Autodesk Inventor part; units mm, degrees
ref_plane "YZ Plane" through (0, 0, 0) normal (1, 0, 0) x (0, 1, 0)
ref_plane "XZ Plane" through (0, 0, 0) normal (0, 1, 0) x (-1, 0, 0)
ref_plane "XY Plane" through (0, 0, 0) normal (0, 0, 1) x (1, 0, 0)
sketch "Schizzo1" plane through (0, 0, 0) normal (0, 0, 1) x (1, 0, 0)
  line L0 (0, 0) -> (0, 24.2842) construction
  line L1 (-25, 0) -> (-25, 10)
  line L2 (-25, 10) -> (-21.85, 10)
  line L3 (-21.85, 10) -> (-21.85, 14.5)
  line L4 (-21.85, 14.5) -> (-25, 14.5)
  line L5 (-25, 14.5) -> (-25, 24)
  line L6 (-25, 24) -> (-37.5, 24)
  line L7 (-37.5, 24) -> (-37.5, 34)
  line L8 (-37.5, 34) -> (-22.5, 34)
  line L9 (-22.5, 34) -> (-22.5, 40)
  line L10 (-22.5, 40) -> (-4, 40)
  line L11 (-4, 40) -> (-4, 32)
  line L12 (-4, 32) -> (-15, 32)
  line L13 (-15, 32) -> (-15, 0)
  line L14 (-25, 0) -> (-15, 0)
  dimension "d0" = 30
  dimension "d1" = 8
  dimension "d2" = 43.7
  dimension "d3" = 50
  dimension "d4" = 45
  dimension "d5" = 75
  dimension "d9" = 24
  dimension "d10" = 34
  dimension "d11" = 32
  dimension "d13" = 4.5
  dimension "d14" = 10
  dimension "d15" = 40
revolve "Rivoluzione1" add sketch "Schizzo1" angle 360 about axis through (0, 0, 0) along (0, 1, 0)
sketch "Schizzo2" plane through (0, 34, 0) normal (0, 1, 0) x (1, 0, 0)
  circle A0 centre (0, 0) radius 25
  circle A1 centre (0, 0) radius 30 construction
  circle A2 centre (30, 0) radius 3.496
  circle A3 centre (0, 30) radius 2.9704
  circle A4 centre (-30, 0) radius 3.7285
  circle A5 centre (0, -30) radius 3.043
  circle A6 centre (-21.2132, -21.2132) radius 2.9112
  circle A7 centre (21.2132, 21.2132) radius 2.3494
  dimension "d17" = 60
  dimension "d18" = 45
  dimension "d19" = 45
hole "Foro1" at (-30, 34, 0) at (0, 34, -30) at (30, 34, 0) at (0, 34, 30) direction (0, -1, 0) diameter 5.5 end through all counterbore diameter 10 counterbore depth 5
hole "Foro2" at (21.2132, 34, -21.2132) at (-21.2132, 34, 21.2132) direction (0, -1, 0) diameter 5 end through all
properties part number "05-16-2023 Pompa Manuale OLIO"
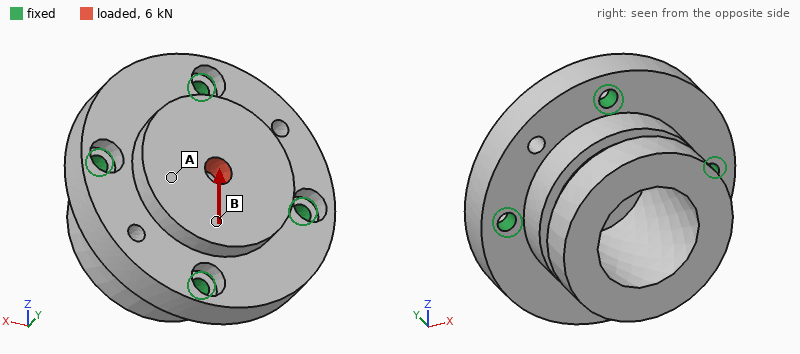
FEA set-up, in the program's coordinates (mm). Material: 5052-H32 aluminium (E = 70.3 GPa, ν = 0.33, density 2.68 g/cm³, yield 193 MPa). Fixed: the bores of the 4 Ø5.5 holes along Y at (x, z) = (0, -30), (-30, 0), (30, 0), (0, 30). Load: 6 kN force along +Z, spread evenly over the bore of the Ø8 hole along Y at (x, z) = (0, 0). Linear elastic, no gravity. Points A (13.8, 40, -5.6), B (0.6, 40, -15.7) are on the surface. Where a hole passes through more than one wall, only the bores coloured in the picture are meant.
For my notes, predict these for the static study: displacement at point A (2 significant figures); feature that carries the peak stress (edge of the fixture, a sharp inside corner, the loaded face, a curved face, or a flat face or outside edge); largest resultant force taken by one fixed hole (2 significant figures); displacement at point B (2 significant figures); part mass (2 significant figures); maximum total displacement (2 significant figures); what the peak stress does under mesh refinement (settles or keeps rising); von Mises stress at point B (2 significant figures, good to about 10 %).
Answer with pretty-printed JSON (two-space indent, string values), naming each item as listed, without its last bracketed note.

{
  "displacement at point A": "5.2 µm",
  "feature that carries the peak stress": "edge of the fixture",
  "largest resultant force taken by one fixed hole": "2.1 kN",
  "displacement at point B": "6.8 µm",
  "part mass": "200 g",
  "maximum total displacement": "9.8 µm",
  "what the peak stress does under mesh refinement": "keeps rising",
  "von Mises stress at point B": "14 MPa"
}
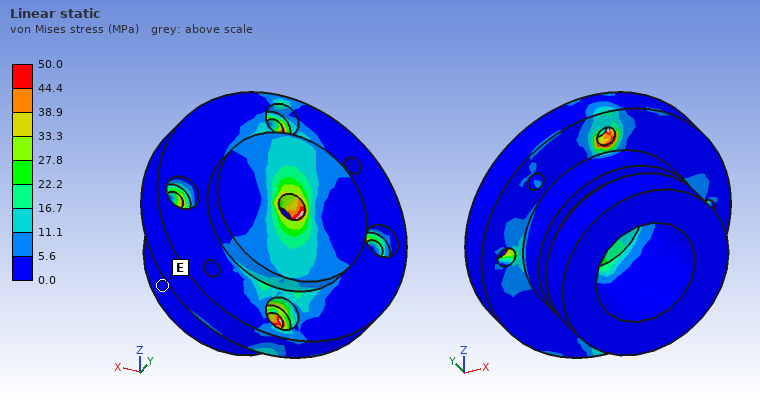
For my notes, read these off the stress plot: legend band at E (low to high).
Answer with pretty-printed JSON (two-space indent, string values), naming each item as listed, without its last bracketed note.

{
  "legend band at E": "0.0 to 5.6 MPa"
}
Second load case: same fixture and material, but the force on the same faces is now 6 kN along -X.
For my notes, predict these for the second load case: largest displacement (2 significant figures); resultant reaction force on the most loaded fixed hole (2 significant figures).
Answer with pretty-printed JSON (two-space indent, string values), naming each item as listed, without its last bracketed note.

{
  "largest displacement": "9.8 µm",
  "resultant reaction force on the most loaded fixed hole": "2.1 kN"
}
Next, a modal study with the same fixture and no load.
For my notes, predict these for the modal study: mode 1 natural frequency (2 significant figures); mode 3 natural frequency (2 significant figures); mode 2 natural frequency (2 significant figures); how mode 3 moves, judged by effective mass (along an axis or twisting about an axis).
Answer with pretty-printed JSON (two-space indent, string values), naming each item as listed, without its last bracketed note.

{
  "mode 1 natural frequency": "12 kHz",
  "mode 3 natural frequency": "13 kHz",
  "mode 2 natural frequency": "12 kHz",
  "how mode 3 moves, judged by effective mass": "along Y"
}
